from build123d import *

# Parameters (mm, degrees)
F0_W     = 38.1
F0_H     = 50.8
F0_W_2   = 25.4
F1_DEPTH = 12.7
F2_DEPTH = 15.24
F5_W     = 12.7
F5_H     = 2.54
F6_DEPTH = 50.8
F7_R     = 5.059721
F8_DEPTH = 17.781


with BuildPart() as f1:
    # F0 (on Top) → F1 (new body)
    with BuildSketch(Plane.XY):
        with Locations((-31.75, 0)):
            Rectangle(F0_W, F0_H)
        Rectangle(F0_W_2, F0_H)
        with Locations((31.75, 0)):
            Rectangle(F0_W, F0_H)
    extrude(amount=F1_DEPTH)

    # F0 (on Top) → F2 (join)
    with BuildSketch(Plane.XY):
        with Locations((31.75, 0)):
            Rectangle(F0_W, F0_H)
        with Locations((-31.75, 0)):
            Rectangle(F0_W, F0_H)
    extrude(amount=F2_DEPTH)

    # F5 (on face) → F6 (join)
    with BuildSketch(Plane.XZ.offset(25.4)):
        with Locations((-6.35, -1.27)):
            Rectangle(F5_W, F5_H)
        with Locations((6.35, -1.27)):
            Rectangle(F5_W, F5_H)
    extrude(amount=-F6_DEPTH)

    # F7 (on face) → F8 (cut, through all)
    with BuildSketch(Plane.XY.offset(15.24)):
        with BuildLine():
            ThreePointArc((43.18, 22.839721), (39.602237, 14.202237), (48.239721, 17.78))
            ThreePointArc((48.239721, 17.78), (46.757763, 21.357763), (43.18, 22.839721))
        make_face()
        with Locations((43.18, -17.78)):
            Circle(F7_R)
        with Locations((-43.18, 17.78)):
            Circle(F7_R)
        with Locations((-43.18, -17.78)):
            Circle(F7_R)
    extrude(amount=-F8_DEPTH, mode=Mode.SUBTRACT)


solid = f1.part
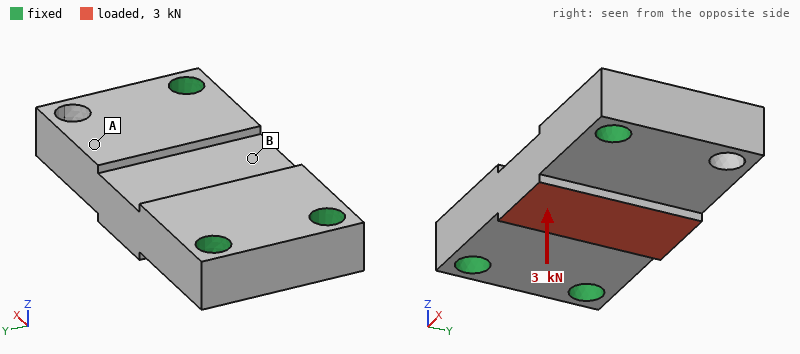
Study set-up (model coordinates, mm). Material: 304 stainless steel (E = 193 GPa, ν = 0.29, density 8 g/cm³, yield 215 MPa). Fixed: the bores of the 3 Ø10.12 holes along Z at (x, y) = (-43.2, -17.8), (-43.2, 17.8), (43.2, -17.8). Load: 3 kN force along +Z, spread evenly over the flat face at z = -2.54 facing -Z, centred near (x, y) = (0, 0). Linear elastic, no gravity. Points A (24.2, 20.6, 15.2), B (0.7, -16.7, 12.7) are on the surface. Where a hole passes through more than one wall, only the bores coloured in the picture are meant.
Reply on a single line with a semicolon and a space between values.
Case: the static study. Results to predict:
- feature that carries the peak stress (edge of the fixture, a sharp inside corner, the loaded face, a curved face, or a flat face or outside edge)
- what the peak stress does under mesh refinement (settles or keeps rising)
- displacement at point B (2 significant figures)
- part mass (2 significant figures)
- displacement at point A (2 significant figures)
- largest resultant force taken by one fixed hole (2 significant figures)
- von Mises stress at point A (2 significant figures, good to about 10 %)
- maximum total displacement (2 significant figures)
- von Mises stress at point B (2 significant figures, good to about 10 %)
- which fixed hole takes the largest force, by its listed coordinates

edge of the fixture; keeps rising; 4.1 µm; 590 g; 6.1 µm; 1.4 kN; 4.2 MPa; 7.7 µm; 11 MPa; (43.2, -17.8)
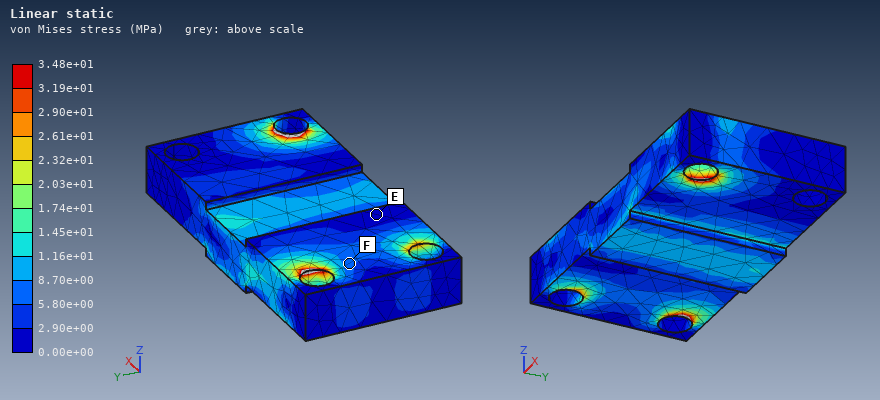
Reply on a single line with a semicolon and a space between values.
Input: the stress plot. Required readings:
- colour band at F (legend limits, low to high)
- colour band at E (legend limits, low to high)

5.80e+00 to 8.70e+00 MPa; 0.00e+00 to 2.90e+00 MPa
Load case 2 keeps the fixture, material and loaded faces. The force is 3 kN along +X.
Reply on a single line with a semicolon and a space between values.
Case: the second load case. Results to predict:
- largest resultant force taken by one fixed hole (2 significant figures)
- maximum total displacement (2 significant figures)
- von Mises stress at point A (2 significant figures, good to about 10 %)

1.2 kN; 2.2 µm; 2.4 MPa
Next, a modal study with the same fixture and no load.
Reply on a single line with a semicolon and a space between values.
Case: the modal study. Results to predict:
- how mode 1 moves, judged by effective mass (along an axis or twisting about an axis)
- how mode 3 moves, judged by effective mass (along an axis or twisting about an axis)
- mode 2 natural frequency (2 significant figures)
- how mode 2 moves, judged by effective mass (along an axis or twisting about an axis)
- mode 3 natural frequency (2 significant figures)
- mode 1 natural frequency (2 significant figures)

along Z; along Y; 9800 Hz; along Z; 13 kHz; 6100 Hz
